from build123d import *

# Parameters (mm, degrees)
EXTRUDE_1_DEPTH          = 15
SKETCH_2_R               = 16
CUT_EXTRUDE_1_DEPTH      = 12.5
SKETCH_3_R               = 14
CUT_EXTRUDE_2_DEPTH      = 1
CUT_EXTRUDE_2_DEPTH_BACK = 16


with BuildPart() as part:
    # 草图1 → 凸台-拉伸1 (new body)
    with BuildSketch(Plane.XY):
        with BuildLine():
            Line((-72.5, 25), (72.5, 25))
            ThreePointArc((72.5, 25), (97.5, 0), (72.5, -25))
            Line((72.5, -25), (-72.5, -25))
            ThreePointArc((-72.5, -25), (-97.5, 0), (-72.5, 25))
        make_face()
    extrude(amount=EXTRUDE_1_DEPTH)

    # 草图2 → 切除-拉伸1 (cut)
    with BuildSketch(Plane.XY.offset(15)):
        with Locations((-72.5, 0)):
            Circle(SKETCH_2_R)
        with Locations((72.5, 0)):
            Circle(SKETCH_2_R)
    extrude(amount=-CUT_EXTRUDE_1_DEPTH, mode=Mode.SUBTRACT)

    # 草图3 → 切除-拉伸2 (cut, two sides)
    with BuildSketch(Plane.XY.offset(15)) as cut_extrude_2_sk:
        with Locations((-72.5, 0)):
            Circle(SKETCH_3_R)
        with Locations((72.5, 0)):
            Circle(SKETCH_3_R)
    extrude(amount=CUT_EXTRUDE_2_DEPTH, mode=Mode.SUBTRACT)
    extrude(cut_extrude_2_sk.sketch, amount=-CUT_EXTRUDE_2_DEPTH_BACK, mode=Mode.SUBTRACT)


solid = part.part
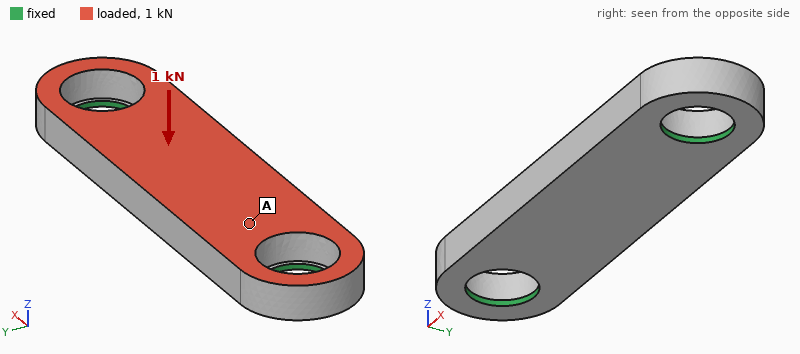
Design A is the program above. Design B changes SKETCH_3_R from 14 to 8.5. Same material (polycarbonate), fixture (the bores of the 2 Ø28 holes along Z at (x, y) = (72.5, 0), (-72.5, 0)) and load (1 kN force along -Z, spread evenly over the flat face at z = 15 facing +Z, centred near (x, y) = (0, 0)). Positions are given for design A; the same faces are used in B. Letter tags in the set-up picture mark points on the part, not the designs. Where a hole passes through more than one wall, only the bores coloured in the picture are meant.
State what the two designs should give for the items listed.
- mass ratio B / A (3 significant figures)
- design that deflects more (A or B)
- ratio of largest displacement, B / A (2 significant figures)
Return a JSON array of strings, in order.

["1.02", "B", "2.2"]
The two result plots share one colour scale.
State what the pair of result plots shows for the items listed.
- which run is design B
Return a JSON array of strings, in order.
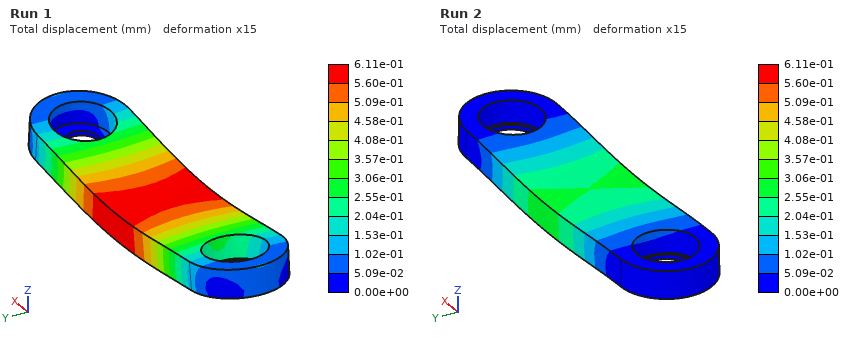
["Run 1"]
